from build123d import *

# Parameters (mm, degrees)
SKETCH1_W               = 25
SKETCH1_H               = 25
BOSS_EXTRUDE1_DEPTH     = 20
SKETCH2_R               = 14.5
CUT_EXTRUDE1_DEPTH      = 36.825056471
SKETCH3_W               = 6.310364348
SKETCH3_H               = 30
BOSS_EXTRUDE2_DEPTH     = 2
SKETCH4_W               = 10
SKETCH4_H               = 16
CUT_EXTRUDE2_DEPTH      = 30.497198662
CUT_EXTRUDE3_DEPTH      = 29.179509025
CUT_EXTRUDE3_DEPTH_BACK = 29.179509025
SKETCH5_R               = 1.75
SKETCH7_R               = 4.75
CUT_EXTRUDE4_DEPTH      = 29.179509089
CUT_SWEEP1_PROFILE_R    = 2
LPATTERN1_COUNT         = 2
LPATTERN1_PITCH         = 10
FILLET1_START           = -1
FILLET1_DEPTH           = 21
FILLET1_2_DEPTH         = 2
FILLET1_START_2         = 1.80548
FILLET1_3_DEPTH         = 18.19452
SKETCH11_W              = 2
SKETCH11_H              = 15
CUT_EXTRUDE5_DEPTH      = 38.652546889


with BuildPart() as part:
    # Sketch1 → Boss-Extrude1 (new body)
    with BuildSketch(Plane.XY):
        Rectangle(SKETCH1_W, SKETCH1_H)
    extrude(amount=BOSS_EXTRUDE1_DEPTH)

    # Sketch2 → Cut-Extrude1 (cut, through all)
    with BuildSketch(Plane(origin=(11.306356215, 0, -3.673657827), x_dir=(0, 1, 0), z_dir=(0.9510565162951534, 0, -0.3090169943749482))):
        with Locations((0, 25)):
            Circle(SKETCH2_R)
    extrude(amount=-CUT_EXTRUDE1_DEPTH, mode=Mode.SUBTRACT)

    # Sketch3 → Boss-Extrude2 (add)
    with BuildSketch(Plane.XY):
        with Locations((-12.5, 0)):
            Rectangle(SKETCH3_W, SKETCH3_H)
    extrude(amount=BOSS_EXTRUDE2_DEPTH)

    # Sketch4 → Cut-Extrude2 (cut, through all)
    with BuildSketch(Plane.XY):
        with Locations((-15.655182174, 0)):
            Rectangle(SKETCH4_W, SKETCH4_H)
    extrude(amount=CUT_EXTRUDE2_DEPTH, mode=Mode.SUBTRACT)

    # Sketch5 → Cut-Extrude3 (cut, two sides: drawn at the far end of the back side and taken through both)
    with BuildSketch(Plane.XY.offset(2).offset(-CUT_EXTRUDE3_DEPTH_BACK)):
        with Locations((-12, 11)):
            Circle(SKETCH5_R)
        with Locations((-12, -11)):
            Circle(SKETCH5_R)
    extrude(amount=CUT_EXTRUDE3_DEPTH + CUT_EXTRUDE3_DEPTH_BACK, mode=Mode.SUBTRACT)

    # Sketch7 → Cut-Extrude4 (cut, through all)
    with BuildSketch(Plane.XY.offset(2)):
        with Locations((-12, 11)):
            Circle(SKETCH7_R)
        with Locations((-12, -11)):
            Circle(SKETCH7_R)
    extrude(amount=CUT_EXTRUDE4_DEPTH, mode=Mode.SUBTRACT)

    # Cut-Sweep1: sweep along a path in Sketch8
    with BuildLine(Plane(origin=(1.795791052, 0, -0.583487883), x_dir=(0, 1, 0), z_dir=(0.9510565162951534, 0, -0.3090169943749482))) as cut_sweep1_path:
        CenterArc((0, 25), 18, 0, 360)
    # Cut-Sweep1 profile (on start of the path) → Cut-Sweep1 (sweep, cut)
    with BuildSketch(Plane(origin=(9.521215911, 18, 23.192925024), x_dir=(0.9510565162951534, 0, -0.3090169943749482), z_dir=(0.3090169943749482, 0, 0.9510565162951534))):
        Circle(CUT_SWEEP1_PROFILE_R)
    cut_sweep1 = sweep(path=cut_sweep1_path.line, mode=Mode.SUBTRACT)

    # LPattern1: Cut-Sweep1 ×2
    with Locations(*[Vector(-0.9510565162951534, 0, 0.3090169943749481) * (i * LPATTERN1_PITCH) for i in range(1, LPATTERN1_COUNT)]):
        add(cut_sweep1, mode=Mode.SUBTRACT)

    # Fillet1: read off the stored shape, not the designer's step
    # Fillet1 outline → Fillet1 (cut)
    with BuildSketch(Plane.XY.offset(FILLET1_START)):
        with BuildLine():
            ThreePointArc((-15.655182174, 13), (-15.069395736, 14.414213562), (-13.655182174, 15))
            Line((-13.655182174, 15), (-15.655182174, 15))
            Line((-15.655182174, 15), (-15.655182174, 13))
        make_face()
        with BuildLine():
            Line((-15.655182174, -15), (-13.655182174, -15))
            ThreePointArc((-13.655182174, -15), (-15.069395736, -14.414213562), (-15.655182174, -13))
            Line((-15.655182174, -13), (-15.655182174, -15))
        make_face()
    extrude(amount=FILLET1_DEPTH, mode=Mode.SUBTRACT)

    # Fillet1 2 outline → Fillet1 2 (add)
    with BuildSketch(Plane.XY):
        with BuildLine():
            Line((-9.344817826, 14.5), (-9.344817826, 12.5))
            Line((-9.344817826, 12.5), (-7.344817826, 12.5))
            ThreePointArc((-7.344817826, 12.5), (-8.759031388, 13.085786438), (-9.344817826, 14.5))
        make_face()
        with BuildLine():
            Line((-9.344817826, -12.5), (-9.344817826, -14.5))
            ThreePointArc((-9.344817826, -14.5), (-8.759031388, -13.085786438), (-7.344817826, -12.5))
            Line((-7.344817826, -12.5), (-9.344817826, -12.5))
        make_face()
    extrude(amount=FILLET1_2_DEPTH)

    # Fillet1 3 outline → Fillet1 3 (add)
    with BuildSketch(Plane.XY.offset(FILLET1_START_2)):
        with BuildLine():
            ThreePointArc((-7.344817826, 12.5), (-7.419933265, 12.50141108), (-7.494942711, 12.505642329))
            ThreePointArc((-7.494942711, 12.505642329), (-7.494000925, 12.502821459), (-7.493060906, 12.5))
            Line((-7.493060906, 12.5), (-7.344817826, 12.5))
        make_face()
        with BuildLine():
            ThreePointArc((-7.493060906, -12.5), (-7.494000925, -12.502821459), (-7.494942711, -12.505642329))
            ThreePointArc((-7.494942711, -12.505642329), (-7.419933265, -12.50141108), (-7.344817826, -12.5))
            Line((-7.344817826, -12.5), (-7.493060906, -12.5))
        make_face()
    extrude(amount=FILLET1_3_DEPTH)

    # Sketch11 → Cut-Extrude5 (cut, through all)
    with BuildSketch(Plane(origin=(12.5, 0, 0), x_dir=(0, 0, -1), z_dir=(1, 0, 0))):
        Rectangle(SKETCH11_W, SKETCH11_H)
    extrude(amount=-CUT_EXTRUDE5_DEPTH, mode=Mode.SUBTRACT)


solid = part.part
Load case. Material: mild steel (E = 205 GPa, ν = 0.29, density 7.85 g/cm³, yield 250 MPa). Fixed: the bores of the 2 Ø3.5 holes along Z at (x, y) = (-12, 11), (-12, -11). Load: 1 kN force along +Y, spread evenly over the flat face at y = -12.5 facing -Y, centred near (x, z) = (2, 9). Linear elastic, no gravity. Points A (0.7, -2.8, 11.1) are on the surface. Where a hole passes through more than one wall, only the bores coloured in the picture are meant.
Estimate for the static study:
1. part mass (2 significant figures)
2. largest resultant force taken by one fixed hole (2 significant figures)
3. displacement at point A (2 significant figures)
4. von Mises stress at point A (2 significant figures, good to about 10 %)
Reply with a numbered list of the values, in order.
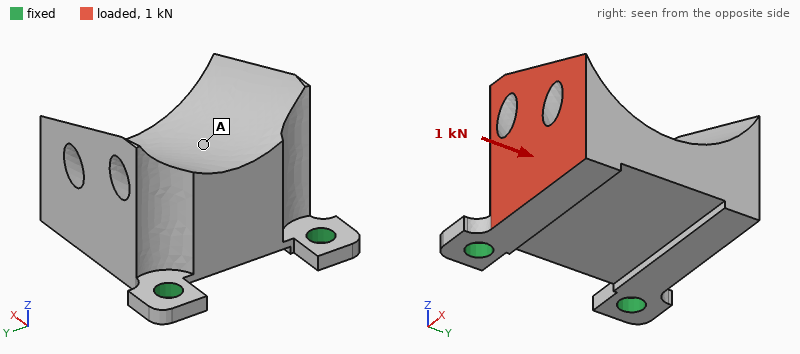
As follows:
1. 47 g
2. 840 N
3. 6.6 µm
4. 15 MPa
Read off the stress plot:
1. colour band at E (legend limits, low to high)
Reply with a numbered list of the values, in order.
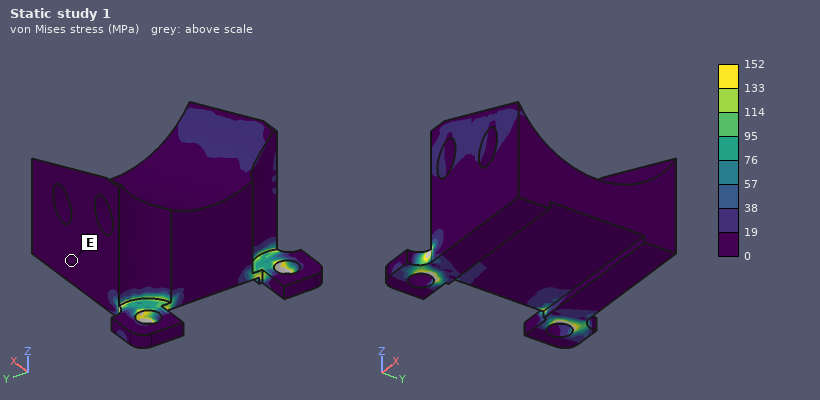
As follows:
1. 0 to 19 MPa
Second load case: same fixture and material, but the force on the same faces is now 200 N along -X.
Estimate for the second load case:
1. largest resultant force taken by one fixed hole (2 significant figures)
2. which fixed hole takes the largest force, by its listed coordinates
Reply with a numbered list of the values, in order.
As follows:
1. 240 N
2. (-12, -11)
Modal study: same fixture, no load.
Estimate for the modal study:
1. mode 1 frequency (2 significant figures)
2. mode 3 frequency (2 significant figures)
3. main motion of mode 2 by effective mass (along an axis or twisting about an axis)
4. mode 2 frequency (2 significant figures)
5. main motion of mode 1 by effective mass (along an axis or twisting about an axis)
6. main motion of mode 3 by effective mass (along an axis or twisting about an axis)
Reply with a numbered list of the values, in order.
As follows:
1. 1200 Hz
2. 12 kHz
3. along Y
4. 8900 Hz
5. along Z
6. along Y
